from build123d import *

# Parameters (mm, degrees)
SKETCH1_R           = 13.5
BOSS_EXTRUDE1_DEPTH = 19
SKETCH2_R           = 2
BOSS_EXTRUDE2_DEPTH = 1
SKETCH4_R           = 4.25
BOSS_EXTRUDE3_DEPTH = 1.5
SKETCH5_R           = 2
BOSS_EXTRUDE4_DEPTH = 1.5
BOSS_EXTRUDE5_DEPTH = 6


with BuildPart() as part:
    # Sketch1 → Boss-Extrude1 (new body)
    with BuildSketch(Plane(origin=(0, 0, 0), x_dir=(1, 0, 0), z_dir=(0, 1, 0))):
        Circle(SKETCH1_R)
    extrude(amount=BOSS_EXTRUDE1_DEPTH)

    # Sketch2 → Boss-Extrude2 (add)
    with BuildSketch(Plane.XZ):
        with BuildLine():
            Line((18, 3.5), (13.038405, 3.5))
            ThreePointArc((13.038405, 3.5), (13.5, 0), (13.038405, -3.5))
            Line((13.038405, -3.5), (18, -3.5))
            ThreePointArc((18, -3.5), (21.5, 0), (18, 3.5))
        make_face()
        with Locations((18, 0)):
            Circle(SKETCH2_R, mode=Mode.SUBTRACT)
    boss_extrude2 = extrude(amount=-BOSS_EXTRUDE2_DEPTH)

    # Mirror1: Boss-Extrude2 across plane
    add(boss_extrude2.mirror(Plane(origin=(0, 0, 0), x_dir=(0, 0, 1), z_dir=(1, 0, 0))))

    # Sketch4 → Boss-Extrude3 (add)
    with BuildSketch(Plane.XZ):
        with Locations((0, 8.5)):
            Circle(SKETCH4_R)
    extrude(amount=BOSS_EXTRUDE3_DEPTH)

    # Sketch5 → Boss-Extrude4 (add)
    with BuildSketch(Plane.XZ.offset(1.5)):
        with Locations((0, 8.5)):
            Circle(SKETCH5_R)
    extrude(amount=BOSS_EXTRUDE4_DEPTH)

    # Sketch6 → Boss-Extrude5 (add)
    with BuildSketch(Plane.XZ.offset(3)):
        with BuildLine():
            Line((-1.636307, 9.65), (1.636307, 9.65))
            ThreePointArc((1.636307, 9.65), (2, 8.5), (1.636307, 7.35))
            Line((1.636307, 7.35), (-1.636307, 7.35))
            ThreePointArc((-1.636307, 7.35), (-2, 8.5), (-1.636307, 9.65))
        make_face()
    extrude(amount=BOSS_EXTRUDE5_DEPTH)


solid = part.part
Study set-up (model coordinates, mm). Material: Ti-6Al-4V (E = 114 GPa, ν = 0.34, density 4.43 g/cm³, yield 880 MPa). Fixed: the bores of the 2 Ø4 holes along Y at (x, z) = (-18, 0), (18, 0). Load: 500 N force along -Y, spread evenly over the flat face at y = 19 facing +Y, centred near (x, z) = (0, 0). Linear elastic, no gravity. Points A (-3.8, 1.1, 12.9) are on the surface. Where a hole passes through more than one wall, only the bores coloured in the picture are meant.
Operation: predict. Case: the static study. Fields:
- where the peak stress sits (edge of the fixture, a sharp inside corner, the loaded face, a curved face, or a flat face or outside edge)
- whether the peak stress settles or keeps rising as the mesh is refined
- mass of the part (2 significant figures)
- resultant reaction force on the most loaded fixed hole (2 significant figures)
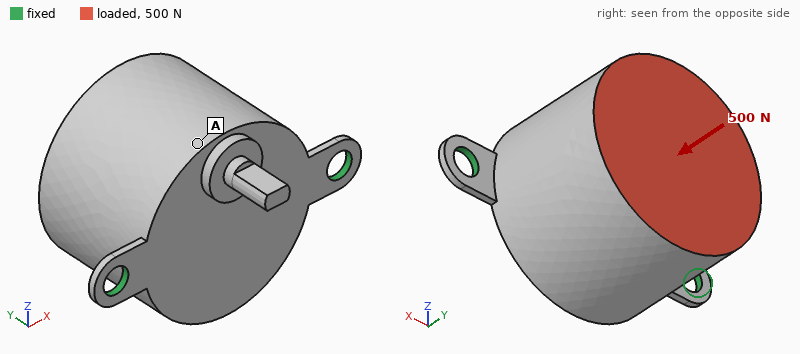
edge of the fixture
keeps rising
49 g
290 N
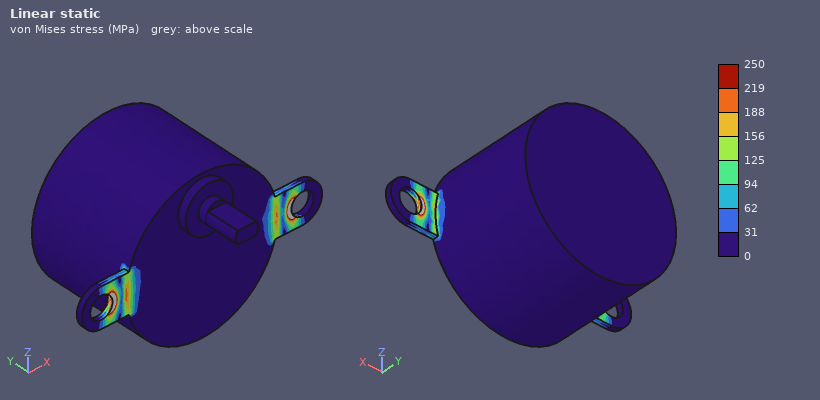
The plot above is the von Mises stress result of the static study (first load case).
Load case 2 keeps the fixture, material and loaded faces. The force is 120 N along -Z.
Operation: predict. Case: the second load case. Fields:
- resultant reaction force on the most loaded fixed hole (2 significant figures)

60 N
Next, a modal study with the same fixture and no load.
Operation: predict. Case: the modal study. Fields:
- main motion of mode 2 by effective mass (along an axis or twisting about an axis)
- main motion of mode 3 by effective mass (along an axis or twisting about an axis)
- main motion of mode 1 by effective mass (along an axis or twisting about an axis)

along Y
along X
along Z
